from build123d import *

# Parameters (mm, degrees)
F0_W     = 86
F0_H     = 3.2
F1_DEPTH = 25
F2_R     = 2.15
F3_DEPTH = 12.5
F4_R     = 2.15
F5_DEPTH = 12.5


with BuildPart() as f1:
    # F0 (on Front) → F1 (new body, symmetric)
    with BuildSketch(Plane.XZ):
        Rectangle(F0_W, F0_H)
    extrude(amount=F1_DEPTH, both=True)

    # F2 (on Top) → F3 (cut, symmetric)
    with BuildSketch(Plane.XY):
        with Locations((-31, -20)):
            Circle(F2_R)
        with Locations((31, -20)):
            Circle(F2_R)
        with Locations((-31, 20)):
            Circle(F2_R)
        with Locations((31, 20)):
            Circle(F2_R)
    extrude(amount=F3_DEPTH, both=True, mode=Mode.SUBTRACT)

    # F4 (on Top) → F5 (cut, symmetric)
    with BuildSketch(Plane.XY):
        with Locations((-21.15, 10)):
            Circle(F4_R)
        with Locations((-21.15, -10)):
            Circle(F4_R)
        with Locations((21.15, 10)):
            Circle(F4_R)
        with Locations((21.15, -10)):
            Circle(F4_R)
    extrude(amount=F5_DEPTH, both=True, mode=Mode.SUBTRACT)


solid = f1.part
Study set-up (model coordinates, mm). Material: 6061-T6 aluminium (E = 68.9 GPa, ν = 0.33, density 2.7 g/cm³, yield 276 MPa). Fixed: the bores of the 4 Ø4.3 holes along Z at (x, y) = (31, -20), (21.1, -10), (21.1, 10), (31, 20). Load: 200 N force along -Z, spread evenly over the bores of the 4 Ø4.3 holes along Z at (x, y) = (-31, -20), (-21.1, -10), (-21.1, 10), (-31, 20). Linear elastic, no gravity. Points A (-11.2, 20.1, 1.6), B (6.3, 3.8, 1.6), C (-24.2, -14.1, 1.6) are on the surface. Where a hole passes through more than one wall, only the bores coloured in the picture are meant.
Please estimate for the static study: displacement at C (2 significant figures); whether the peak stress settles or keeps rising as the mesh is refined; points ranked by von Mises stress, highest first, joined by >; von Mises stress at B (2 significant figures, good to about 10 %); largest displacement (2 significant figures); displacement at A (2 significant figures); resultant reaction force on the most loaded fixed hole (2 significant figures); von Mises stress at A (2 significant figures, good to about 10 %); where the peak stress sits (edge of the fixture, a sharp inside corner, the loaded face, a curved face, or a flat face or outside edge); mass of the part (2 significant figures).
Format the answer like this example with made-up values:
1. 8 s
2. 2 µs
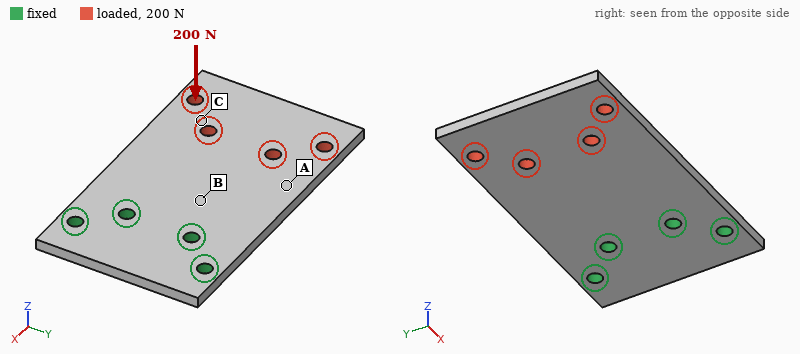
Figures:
1. 0.66 mm
2. keeps rising
3. B > A > C
4. 69 MPa
5. 1.1 mm
6. 0.37 mm
7. 240 N
8. 36 MPa
9. edge of the fixture
10. 36 g
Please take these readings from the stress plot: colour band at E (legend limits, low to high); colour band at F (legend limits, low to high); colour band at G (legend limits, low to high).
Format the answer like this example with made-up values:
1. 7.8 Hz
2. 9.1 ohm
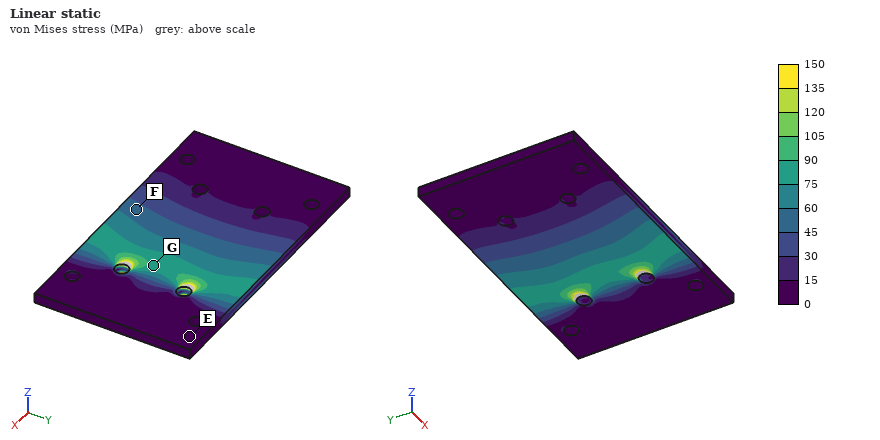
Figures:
1. 0 to 15 MPa
2. 45 to 60 MPa
3. 75 to 90 MPa
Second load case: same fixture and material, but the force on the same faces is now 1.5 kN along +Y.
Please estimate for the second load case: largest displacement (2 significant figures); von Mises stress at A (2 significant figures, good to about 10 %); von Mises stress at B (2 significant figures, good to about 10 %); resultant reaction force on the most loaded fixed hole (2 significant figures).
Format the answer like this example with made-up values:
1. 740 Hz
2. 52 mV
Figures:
1. 74 µm
2. 16 MPa
3. 28 MPa
4. 1.4 kN
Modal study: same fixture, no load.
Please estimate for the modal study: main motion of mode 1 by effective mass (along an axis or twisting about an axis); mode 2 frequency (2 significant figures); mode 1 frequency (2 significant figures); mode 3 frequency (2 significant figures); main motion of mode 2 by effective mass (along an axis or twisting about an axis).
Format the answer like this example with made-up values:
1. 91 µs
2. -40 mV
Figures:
1. along Z
2. 1800 Hz
3. 660 Hz
4. 3900 Hz
5. twisting about X
